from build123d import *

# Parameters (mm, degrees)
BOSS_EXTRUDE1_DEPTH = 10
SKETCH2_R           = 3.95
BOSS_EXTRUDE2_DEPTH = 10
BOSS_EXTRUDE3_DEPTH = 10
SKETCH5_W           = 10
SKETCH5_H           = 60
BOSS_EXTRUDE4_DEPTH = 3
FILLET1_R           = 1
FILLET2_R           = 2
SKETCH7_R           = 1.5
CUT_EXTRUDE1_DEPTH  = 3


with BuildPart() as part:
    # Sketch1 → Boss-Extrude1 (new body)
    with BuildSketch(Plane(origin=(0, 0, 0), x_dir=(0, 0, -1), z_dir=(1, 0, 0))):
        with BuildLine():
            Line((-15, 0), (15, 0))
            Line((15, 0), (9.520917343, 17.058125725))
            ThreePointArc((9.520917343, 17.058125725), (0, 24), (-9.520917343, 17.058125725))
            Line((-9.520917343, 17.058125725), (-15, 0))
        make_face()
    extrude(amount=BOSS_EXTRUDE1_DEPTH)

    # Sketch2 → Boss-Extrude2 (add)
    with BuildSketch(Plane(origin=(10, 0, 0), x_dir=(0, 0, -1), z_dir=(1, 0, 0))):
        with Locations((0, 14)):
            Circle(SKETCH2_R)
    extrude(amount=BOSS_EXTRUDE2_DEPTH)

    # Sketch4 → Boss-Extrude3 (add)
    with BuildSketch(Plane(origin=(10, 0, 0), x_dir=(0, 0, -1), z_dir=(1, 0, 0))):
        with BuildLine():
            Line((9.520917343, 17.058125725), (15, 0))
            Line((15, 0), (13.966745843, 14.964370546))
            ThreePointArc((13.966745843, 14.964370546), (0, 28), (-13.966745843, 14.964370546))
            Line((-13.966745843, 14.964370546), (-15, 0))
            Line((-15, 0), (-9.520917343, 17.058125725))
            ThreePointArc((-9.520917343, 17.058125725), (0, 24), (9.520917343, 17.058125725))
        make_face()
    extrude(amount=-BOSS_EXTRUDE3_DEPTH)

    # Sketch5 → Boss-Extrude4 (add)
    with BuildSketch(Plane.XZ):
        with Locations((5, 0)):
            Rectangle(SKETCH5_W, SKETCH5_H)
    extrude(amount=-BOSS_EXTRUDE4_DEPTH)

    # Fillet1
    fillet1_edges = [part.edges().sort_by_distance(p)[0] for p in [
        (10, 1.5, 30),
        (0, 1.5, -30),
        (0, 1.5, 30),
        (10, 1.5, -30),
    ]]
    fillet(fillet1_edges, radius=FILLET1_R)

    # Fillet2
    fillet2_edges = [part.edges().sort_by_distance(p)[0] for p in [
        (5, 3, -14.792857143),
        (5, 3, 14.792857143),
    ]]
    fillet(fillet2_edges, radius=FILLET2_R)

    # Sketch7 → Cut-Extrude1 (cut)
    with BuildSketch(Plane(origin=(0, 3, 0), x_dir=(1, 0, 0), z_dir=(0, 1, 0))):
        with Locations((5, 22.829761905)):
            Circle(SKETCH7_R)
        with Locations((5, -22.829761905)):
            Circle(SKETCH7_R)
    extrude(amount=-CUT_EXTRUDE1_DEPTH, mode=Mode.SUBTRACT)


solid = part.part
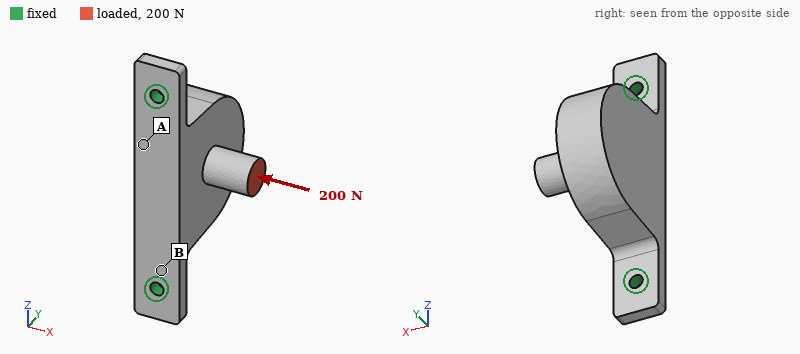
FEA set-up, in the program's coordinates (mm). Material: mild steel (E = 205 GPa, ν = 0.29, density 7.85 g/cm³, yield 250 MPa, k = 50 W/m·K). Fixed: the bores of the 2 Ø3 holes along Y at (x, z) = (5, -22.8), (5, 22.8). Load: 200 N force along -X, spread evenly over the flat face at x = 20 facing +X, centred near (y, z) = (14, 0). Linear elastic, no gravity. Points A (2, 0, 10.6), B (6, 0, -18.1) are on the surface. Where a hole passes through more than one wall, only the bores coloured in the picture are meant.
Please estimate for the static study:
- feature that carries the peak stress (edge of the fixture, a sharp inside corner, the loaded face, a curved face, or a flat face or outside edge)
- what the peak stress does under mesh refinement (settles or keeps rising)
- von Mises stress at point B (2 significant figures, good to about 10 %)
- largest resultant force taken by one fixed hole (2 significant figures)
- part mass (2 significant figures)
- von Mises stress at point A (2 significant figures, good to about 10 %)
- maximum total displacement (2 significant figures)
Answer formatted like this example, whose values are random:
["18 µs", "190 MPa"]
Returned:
["edge of the fixture", "keeps rising", "52 MPa", "100 N", "67 g", "13 MPa", "39 µm"]
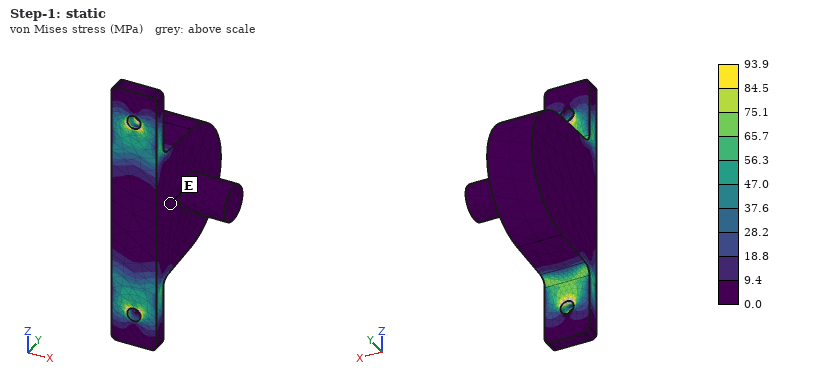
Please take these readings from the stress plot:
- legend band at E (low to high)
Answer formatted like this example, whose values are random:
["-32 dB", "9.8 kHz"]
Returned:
["0.0 to 9.4 MPa"]
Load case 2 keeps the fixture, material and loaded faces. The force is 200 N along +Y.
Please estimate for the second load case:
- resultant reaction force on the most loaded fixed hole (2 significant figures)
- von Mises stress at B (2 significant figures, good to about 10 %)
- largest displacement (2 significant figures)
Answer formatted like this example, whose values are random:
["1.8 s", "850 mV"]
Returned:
["120 N", "72 MPa", "46 µm"]
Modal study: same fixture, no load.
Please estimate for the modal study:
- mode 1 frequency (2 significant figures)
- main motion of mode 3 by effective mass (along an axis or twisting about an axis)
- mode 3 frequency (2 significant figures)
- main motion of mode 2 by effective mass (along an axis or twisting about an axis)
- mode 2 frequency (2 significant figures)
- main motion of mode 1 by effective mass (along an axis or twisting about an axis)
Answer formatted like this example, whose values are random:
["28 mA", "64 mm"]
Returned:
["1900 Hz", "along Z", "8500 Hz", "along Y", "7100 Hz", "along X"]
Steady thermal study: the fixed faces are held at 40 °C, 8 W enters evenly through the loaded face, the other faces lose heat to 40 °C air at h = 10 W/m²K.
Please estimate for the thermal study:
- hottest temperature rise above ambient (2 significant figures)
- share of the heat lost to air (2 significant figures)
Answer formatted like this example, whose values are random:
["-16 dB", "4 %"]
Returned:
["70 K", "10 %"]
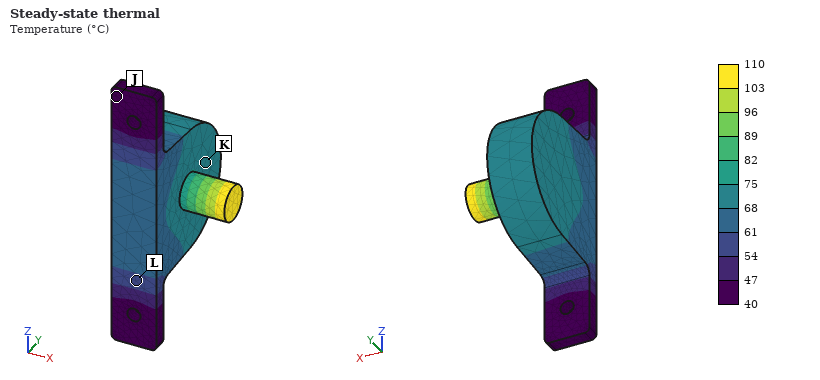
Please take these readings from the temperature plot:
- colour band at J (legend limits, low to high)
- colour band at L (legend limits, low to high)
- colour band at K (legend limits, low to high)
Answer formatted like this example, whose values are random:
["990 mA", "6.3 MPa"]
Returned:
["40 to 47 °C", "54 to 61 °C", "68 to 75 °C"]
